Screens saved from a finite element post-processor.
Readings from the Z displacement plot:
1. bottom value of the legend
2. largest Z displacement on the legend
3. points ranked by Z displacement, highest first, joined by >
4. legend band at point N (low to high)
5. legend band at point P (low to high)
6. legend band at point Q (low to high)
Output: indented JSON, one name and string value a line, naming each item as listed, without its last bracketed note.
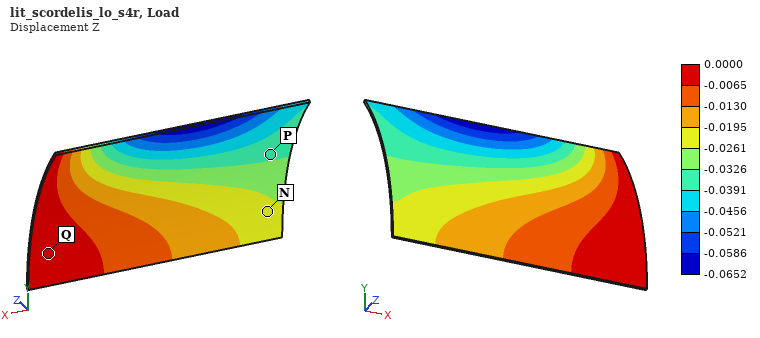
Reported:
{
  "bottom value of the legend": "-0.0652",
  "largest Z displacement on the legend": "0.0000",
  "points ranked by Z displacement, highest first, joined by >": "Q > N > P",
  "legend band at point N": "-0.0261 to -0.0195",
  "legend band at point P": "-0.0391 to -0.0326",
  "legend band at point Q": "-0.0065 to 0.0000"
}
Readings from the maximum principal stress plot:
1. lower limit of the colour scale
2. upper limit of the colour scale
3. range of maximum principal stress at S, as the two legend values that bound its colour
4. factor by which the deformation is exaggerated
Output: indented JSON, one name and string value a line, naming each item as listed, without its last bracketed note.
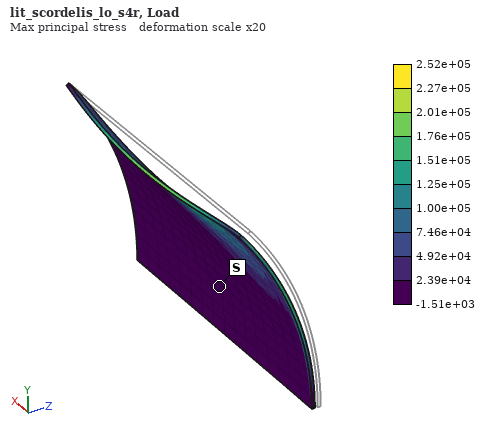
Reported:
{
  "lower limit of the colour scale": "-1.51e+03",
  "upper limit of the colour scale": "2.52e+05",
  "range of maximum principal stress at S, as the two legend values that bound its colour": "-1.51e+03 to 2.39e+04",
  "factor by which the deformation is exaggerated": "20"
}
